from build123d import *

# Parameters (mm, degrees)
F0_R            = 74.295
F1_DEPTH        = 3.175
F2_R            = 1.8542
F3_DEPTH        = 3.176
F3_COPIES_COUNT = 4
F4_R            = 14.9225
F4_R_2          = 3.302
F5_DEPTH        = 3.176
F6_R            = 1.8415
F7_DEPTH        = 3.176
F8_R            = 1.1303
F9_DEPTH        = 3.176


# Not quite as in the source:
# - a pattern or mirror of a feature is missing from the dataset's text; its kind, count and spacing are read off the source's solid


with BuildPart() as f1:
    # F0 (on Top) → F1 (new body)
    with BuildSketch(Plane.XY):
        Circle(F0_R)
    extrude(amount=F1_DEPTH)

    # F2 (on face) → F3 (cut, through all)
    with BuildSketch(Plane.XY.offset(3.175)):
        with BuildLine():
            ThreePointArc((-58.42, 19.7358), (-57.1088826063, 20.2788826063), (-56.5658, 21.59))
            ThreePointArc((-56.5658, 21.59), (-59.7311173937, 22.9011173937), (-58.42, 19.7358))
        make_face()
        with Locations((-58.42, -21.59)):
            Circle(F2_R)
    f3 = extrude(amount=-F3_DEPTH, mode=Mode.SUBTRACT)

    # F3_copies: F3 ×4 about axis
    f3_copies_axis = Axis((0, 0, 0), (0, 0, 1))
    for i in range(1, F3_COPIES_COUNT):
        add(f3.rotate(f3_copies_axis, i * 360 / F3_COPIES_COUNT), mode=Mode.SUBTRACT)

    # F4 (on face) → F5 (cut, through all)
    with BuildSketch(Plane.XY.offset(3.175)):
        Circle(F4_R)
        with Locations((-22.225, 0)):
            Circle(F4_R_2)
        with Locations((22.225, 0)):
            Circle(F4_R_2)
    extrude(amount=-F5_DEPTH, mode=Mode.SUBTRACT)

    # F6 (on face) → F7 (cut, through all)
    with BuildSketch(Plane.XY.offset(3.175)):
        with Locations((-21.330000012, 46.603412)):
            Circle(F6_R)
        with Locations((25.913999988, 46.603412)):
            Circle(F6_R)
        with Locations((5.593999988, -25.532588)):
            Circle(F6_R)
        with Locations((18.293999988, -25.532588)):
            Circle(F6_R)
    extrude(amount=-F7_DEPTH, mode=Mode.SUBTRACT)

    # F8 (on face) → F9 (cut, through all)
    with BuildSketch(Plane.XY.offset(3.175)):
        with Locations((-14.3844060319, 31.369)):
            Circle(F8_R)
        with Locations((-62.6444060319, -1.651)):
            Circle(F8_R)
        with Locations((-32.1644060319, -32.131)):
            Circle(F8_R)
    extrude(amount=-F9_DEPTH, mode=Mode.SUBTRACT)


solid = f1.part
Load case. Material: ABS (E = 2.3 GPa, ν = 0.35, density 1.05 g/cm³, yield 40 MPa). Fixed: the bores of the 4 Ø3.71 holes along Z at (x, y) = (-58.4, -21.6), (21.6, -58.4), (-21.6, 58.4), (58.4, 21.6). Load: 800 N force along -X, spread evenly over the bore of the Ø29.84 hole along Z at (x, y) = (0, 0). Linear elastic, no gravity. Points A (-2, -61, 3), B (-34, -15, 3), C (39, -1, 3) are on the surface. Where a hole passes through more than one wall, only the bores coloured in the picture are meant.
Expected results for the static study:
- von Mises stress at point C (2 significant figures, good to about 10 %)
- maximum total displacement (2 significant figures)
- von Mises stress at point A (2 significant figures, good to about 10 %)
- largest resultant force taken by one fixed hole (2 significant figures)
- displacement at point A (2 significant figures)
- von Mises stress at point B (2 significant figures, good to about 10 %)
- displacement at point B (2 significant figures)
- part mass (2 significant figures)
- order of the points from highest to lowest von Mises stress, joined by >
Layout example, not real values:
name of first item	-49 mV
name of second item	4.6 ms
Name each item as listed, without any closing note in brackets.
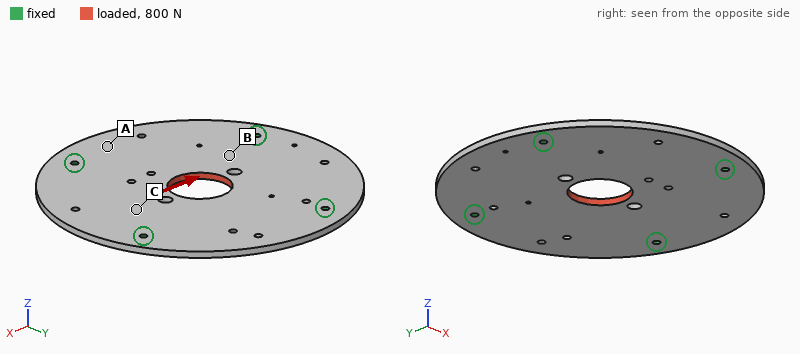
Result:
von Mises stress at point C	1.8 MPa
maximum total displacement	82 µm
von Mises stress at point A	0.70 MPa
largest resultant force taken by one fixed hole	240 N
displacement at point A	15 µm
von Mises stress at point B	2.9 MPa
displacement at point B	40 µm
part mass	55 g
order of the points from highest to lowest von Mises stress, joined by >	B > C > A
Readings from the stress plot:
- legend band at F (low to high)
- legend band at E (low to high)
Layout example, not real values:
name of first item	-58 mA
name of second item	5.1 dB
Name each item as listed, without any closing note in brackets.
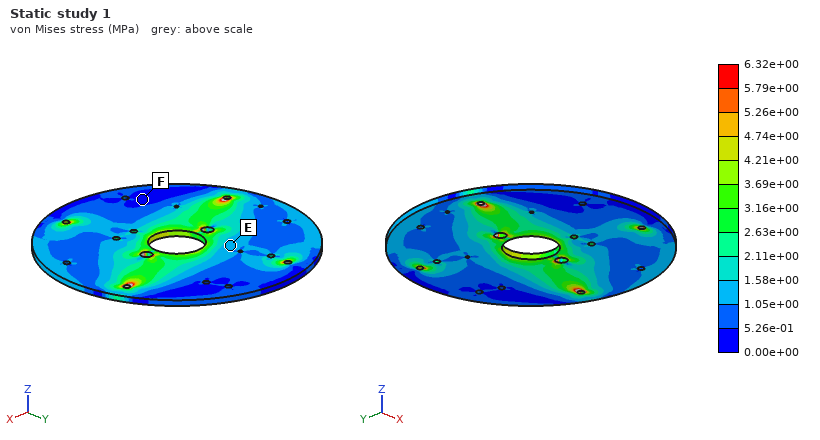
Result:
legend band at F	0.00e+00 to 5.26e-01 MPa
legend band at E	1.05e+00 to 1.58e+00 MPa
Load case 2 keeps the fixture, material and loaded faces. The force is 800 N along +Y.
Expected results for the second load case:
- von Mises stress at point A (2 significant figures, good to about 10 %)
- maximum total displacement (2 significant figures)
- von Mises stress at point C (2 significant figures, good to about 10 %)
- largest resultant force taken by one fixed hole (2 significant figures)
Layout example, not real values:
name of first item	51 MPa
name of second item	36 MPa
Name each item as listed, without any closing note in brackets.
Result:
von Mises stress at point A	0.92 MPa
maximum total displacement	76 µm
von Mises stress at point C	1.1 MPa
largest resultant force taken by one fixed hole	240 N
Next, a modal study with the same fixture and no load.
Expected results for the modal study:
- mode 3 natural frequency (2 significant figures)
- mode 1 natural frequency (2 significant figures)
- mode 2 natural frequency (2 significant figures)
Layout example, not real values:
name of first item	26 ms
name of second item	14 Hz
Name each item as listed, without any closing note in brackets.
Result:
mode 3 natural frequency	480 Hz
mode 1 natural frequency	430 Hz
mode 2 natural frequency	440 Hz
